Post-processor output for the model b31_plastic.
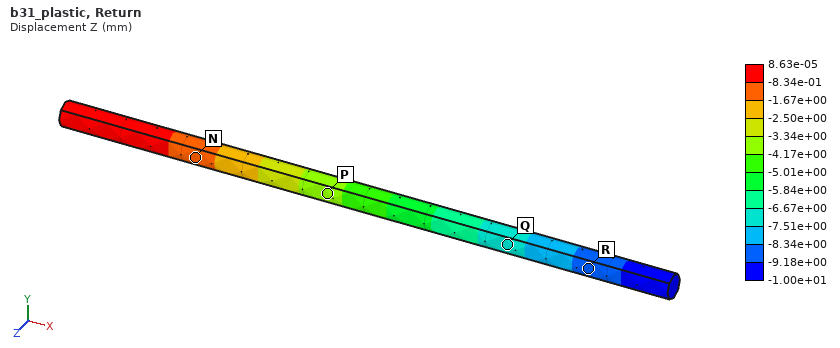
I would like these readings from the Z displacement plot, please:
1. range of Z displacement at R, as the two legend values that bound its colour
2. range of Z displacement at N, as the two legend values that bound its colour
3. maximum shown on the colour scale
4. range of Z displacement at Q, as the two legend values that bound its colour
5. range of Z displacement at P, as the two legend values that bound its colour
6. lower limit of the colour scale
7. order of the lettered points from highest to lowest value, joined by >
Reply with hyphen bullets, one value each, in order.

- -9.18e+00 to -8.34e+00 mm
- -1.67e+00 to -8.34e-01 mm
- 8.63e-05 mm
- -7.51e+00 to -6.67e+00 mm
- -4.17e+00 to -3.34e+00 mm
- -1.00e+01 mm
- N > P > Q > R
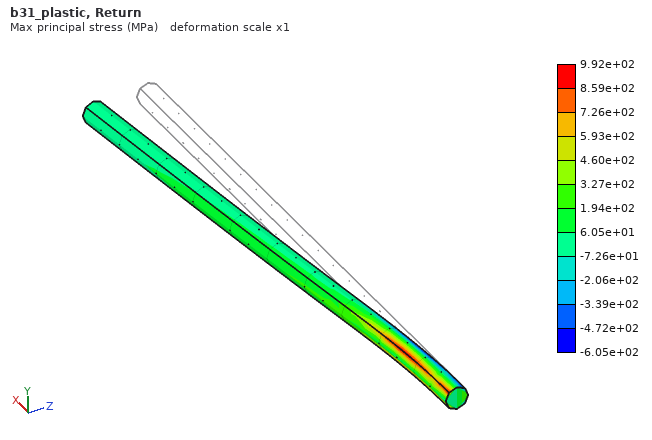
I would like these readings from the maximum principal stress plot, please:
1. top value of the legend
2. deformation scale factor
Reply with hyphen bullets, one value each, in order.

- 9.92e+02 MPa
- 1
